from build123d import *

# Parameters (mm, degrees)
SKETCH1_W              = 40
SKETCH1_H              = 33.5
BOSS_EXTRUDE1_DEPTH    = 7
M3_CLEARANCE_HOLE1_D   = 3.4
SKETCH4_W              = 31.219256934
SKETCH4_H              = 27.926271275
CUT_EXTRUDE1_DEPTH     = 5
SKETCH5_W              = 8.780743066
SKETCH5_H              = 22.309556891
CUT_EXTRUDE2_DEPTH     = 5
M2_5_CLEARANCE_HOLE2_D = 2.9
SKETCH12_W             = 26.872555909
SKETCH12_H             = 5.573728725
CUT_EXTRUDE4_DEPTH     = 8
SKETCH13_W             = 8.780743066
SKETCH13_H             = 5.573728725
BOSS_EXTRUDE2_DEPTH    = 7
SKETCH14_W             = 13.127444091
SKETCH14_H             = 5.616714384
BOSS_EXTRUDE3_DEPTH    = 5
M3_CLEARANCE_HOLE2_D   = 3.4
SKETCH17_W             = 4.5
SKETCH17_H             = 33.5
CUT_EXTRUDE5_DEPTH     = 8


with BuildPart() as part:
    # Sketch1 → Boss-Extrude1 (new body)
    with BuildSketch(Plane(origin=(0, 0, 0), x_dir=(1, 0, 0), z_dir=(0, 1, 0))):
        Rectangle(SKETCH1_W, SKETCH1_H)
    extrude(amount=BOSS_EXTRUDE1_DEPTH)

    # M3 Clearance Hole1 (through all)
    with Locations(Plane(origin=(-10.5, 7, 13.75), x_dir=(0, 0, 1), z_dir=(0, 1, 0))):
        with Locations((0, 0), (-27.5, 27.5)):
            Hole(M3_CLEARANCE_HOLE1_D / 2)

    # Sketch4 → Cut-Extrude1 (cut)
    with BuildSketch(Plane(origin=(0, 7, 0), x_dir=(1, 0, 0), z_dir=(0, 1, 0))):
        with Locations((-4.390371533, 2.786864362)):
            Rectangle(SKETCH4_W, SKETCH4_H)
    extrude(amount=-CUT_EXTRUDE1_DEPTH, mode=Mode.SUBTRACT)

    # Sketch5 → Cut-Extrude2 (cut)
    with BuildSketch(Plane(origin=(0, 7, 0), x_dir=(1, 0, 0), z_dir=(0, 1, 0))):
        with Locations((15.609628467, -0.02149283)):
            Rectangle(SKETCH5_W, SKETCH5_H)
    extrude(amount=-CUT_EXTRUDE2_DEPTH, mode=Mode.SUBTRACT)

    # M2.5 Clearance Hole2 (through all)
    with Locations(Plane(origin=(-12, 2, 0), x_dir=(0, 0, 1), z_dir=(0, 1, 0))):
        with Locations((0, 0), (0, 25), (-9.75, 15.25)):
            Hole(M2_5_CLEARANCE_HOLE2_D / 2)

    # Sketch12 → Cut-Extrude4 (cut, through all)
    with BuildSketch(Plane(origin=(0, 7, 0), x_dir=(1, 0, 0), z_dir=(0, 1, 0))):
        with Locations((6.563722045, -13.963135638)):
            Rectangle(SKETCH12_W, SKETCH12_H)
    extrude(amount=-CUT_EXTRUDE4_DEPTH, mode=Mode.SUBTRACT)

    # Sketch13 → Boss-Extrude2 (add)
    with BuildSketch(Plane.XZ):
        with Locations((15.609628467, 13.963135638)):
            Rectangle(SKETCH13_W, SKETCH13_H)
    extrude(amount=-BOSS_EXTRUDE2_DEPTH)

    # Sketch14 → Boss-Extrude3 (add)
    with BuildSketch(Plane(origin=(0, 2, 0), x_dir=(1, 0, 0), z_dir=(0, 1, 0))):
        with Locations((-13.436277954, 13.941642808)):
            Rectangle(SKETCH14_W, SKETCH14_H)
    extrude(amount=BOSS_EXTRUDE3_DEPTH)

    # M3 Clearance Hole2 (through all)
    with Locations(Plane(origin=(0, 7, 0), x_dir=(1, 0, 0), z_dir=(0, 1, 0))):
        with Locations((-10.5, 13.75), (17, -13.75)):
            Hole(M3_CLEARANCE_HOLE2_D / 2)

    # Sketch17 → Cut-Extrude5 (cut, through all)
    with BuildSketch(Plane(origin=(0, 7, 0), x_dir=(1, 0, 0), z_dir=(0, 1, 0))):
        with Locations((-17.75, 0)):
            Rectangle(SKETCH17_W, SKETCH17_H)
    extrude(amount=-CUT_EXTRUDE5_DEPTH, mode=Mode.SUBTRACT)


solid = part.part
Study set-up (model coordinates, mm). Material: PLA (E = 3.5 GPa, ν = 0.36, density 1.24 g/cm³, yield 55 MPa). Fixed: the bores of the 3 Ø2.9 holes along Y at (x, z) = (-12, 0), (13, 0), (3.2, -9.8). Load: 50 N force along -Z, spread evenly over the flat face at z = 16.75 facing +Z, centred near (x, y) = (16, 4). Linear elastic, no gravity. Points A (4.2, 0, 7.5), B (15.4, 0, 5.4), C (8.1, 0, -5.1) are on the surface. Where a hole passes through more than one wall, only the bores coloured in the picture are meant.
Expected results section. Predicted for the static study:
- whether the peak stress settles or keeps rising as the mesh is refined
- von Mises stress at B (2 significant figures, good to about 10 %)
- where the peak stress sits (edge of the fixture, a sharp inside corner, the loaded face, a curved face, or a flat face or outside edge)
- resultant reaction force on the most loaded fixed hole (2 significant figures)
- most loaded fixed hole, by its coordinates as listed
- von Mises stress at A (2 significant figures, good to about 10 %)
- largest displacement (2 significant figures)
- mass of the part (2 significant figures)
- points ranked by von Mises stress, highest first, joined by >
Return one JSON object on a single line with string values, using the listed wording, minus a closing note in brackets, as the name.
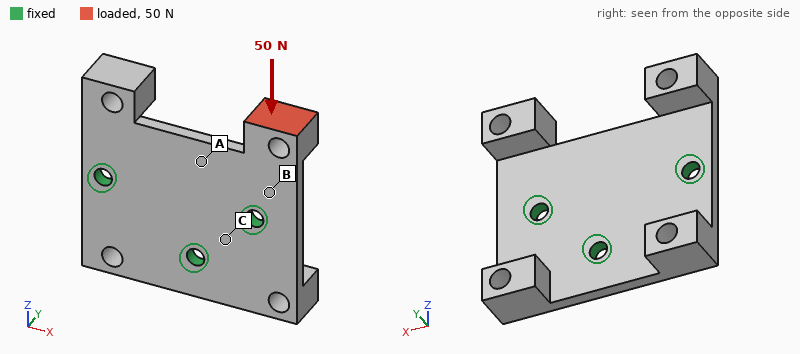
{"whether the peak stress settles or keeps rising as the mesh is refined": "keeps rising", "von Mises stress at B": "9.1 MPa", "where the peak stress sits": "a sharp inside corner", "resultant reaction force on the most loaded fixed hole": "49 N", "most loaded fixed hole, by its coordinates as listed": "(13, 0)", "von Mises stress at A": "5.8 MPa", "largest displacement": "0.57 mm", "mass of the part": "3.5 g", "points ranked by von Mises stress, highest first, joined by >": "B > A > C"}
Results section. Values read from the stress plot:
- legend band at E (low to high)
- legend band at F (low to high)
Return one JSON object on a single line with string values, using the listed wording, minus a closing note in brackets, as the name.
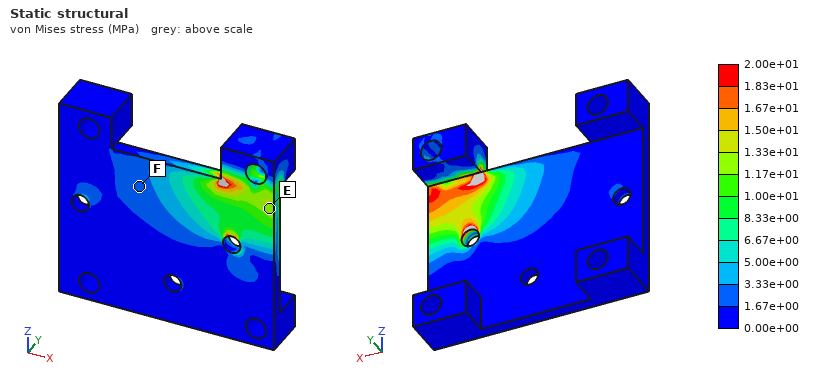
{"legend band at E": "1.17e+01 to 1.33e+01 MPa", "legend band at F": "1.67e+00 to 3.33e+00 MPa"}
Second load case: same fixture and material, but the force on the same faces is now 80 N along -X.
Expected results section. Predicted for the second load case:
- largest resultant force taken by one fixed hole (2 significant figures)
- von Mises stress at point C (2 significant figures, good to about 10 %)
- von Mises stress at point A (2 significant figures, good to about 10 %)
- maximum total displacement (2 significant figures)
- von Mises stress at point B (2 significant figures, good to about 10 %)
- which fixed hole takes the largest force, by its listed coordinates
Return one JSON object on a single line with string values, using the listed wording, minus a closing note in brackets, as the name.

{"largest resultant force taken by one fixed hole": "72 N", "von Mises stress at point C": "2.8 MPa", "von Mises stress at point A": "5.1 MPa", "maximum total displacement": "0.49 mm", "von Mises stress at point B": "18 MPa", "which fixed hole takes the largest force, by its listed coordinates": "(13, 0)"}
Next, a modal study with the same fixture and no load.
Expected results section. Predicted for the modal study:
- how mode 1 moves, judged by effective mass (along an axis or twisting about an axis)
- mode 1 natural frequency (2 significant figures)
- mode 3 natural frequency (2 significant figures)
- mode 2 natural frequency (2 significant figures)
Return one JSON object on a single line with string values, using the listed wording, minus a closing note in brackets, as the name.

{"how mode 1 moves, judged by effective mass": "along Y", "mode 1 natural frequency": "1500 Hz", "mode 3 natural frequency": "2200 Hz", "mode 2 natural frequency": "1600 Hz"}
